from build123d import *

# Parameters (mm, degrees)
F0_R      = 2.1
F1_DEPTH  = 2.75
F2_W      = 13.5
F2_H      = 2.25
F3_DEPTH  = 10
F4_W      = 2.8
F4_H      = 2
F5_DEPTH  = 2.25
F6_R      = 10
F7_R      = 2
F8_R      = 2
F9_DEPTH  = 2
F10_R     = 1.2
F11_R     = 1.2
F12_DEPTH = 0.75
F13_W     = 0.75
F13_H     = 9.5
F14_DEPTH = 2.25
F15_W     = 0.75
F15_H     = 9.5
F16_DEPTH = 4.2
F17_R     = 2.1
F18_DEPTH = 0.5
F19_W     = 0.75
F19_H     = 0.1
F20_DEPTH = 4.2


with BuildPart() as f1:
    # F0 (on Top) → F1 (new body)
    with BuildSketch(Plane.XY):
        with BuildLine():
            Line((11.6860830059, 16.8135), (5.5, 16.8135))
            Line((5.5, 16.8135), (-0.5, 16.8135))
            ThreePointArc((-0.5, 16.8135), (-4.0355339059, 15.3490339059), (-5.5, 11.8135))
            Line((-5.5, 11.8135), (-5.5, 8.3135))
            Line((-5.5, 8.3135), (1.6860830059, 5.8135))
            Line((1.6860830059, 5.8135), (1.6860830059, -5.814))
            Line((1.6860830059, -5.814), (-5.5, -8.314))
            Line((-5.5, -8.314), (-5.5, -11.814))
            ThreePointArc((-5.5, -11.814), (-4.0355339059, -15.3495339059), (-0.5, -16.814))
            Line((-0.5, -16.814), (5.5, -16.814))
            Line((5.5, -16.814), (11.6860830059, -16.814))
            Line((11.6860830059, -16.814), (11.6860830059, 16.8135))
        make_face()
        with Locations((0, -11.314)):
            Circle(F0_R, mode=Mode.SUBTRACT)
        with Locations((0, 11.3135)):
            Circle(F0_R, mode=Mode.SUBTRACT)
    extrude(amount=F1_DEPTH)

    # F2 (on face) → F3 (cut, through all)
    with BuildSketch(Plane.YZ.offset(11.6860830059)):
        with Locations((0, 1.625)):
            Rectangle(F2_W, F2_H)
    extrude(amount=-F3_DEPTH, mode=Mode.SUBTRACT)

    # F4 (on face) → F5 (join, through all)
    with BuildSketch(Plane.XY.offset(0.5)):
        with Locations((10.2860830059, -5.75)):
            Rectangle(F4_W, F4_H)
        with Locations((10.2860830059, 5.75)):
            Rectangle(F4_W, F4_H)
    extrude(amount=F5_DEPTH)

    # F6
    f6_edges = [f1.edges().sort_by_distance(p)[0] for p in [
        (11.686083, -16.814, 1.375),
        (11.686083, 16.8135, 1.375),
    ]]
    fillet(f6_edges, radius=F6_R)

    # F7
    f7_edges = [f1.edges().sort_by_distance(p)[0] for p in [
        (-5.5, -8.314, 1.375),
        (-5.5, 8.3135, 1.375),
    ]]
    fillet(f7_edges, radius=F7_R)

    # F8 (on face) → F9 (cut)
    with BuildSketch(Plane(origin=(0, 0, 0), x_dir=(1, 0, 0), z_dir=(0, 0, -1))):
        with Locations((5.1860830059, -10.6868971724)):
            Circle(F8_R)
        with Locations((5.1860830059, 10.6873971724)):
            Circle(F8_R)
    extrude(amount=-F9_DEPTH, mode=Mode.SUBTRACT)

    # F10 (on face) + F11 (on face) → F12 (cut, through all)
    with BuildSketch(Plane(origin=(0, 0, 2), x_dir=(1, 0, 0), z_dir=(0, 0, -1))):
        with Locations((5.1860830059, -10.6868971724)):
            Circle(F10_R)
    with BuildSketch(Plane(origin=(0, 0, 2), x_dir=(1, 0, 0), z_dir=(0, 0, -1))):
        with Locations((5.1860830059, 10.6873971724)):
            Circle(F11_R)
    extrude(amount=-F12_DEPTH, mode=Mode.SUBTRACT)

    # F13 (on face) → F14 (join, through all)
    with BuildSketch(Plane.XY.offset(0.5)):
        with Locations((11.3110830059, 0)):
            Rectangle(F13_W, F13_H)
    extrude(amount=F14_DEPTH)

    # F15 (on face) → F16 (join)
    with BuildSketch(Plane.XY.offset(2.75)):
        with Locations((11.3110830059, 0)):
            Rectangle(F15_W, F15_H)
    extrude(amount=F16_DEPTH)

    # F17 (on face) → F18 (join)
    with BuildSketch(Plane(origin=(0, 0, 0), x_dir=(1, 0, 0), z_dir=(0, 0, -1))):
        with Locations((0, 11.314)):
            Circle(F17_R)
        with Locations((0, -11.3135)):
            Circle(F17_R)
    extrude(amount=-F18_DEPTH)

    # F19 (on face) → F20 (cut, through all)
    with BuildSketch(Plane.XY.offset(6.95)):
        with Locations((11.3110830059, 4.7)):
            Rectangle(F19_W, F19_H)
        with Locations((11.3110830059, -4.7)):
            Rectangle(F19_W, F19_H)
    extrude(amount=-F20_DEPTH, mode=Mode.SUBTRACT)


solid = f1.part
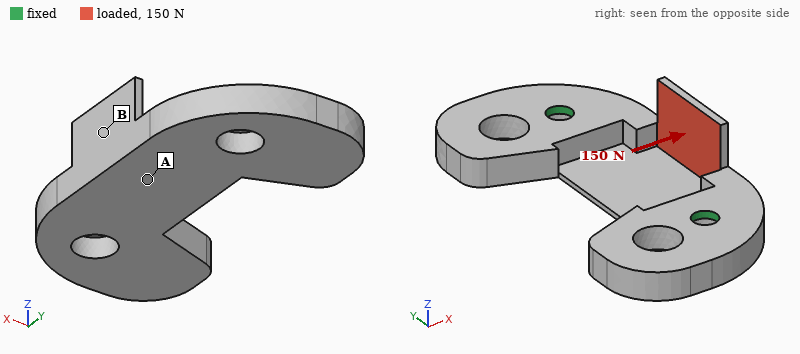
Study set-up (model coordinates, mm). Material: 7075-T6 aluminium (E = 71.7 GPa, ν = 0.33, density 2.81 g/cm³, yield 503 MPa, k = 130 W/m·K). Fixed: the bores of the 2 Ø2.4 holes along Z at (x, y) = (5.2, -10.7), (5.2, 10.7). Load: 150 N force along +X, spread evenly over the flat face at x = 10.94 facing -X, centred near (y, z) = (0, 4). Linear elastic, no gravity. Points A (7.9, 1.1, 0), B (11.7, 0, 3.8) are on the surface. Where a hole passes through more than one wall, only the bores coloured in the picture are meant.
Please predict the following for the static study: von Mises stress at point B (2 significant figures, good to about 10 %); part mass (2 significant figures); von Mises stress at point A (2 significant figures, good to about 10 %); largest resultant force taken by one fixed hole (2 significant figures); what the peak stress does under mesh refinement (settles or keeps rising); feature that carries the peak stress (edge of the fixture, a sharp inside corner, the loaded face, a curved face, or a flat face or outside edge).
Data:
160 MPa
2.3 g
48 MPa
92 N
keeps rising
a sharp inside corner
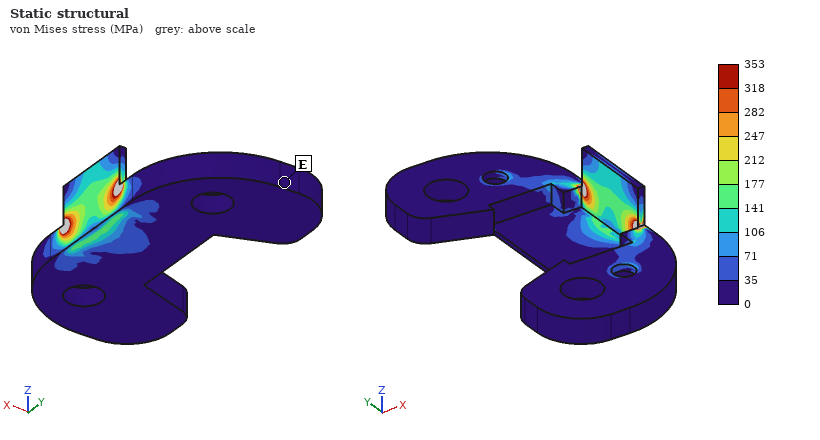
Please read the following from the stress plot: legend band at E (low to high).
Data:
0 to 35 MPa
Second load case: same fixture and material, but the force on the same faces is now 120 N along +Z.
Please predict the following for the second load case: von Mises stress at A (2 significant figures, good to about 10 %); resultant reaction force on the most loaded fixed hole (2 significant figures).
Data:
29 MPa
90 N
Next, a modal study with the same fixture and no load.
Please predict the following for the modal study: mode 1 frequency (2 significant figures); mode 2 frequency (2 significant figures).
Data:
9200 Hz
11 kHz
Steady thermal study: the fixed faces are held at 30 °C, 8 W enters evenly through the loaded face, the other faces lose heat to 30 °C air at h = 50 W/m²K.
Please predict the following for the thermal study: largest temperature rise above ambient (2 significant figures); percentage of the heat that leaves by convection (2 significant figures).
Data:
53 K
7.9 %
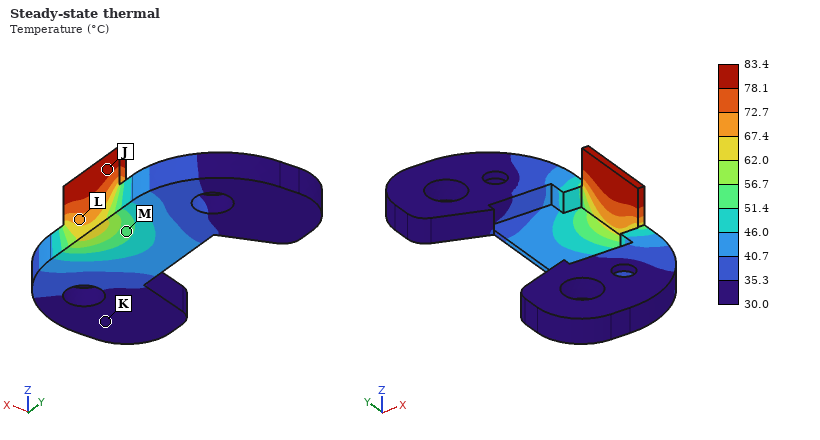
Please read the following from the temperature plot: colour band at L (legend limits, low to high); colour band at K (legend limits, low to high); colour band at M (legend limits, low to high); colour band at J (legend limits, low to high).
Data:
67.4 to 72.7 °C
30.0 to 35.3 °C
51.4 to 56.7 °C
78.1 to 83.4 °C
